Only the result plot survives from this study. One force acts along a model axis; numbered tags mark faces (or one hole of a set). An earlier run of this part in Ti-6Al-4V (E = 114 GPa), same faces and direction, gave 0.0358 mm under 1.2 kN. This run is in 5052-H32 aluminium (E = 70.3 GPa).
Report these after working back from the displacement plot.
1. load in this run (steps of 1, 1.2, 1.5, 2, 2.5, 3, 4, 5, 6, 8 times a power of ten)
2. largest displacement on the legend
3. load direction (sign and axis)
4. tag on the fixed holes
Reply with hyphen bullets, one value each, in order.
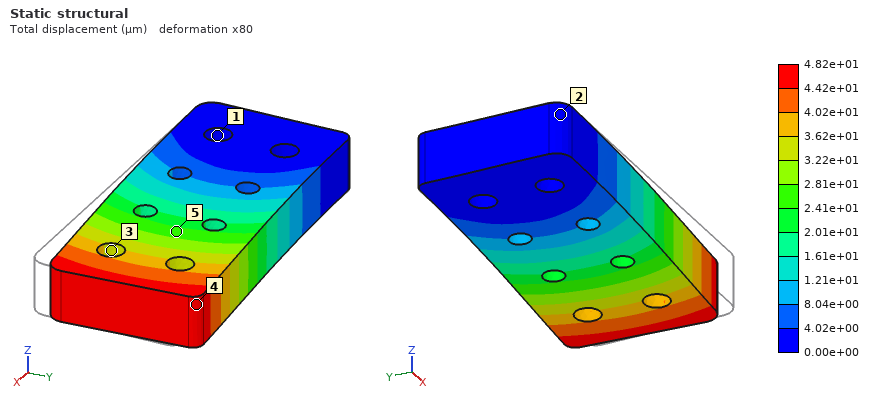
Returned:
- 1 kN
- 4.82e+01 µm
- +Y
- 1
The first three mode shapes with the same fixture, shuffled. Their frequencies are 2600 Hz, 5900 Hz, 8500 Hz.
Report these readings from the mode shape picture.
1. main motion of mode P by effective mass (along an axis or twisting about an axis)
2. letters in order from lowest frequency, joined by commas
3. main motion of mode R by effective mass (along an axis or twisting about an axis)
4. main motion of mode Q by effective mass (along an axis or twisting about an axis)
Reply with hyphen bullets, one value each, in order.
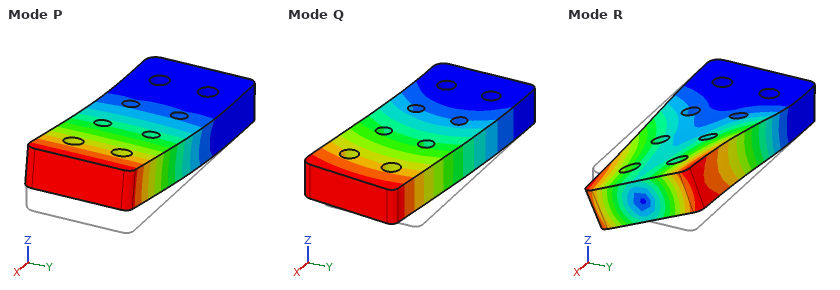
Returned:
- along Z
- P, Q, R
- twisting about X
- along Y
